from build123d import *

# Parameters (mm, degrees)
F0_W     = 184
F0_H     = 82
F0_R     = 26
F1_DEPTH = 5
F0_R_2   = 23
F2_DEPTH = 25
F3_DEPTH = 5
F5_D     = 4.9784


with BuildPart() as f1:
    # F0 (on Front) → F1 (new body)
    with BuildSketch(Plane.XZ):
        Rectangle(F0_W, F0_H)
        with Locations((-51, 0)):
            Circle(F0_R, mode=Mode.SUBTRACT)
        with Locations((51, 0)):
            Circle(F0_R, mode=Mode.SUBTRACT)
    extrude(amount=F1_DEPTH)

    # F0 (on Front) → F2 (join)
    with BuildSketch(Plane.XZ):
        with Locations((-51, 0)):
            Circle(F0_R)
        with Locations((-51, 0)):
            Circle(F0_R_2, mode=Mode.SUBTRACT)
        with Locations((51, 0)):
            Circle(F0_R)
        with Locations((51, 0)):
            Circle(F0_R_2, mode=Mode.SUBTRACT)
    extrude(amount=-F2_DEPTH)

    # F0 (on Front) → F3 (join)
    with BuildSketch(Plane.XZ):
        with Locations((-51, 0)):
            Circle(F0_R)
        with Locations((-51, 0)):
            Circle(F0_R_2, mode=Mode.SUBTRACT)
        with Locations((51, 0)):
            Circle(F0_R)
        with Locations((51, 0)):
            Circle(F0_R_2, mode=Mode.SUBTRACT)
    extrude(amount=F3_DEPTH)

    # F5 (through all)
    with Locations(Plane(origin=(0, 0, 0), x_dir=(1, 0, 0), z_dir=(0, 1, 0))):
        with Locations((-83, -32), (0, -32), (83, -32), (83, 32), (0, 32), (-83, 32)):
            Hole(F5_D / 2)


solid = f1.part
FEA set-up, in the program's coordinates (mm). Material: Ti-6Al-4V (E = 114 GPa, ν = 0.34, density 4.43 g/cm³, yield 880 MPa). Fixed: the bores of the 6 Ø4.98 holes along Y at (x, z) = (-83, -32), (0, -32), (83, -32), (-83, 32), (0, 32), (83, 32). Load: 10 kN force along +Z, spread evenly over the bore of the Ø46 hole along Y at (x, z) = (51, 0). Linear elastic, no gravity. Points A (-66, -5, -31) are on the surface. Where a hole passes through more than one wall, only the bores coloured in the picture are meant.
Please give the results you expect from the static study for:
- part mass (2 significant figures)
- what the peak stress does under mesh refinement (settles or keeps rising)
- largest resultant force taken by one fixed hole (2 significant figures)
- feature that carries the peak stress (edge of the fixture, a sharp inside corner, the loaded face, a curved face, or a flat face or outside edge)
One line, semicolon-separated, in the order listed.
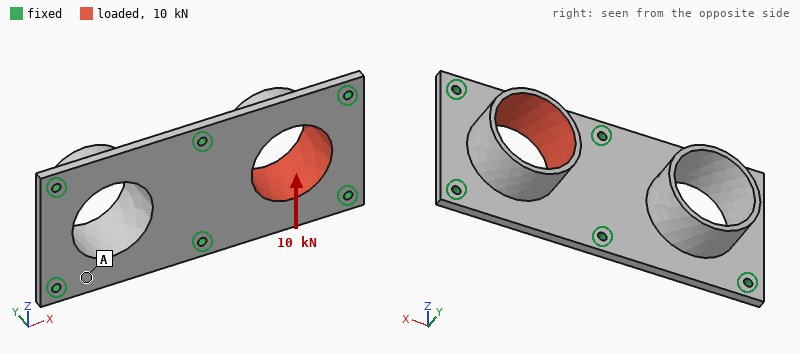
360 g; keeps rising; 3.2 kN; edge of the fixture
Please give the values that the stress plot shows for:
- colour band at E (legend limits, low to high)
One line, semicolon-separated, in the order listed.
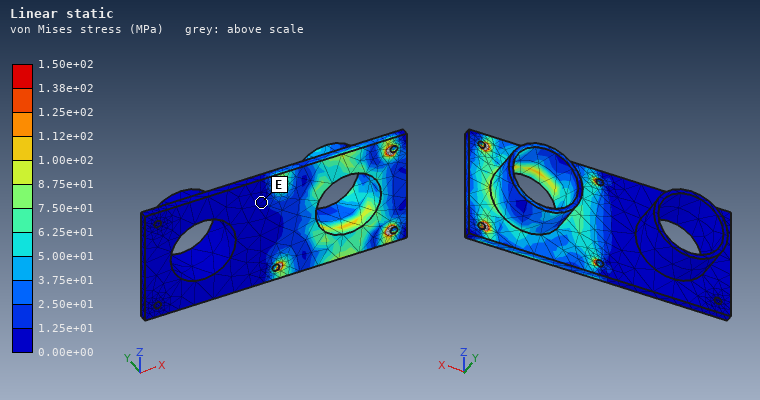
0.00e+00 to 1.25e+01 MPa
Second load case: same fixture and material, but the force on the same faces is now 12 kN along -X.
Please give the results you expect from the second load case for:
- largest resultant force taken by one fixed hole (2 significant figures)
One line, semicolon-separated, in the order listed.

3.4 kN
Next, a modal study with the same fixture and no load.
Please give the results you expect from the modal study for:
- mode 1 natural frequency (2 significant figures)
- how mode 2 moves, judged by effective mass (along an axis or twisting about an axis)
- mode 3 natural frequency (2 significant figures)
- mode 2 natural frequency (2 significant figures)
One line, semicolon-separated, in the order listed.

3100 Hz; along Y; 3900 Hz; 3300 Hz
